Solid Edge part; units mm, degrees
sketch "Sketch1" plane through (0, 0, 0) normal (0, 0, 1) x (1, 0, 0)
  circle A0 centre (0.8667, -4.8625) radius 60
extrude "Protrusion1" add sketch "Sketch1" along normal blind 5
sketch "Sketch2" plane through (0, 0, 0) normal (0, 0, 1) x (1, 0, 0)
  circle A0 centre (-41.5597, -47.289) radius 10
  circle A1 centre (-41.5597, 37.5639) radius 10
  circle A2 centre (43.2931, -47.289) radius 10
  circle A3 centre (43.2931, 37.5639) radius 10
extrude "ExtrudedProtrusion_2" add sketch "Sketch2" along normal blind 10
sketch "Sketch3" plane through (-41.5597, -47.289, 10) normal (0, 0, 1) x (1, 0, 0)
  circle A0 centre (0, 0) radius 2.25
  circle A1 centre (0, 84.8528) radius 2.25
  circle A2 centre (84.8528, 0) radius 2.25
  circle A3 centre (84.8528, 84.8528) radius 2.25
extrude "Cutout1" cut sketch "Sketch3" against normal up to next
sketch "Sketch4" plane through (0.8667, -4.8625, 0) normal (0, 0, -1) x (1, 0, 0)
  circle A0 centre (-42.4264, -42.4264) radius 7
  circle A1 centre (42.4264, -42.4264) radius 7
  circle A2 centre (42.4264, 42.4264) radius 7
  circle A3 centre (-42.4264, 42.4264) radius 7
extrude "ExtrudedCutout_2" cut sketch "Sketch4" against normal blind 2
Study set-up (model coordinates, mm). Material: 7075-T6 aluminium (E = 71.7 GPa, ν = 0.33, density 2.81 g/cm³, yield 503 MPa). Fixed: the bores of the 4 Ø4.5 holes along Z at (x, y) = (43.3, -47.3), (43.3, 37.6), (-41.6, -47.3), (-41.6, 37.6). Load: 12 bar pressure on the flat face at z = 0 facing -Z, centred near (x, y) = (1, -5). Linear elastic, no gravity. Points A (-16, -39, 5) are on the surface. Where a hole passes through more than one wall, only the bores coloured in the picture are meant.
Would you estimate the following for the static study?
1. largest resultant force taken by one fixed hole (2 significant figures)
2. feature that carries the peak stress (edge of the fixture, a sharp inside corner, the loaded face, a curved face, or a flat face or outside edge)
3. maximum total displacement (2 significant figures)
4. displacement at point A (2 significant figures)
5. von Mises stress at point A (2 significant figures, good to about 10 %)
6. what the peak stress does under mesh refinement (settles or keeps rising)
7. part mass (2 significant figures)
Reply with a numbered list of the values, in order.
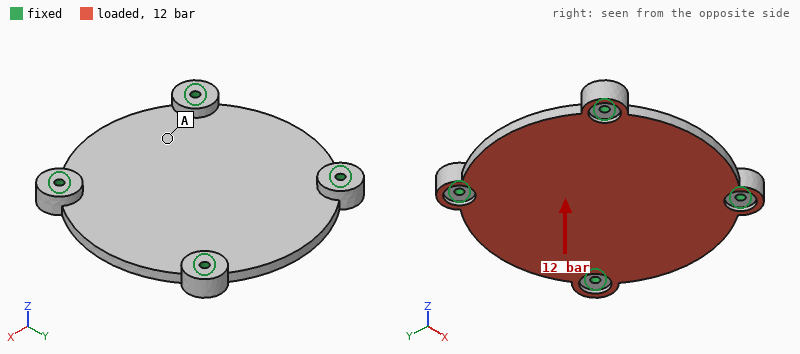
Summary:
1. 5.0 kN
2. edge of the fixture
3. 0.40 mm
4. 0.20 mm
5. 47 MPa
6. keeps rising
7. 180 g
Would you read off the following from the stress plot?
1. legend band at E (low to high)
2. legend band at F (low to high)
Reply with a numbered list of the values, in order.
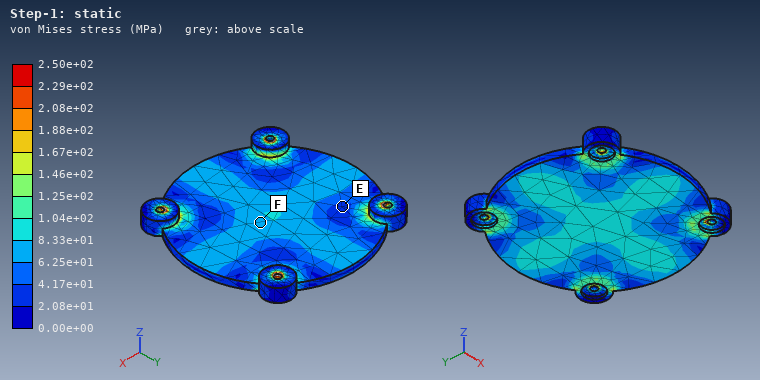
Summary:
1. 2.08e+01 to 4.17e+01 MPa
2. 6.25e+01 to 8.33e+01 MPa
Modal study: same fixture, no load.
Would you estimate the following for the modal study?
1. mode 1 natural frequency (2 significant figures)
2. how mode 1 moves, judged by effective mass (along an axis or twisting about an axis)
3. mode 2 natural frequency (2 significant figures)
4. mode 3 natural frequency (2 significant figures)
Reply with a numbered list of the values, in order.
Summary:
1. 2800 Hz
2. along Z
3. 4000 Hz
4. 4100 Hz
